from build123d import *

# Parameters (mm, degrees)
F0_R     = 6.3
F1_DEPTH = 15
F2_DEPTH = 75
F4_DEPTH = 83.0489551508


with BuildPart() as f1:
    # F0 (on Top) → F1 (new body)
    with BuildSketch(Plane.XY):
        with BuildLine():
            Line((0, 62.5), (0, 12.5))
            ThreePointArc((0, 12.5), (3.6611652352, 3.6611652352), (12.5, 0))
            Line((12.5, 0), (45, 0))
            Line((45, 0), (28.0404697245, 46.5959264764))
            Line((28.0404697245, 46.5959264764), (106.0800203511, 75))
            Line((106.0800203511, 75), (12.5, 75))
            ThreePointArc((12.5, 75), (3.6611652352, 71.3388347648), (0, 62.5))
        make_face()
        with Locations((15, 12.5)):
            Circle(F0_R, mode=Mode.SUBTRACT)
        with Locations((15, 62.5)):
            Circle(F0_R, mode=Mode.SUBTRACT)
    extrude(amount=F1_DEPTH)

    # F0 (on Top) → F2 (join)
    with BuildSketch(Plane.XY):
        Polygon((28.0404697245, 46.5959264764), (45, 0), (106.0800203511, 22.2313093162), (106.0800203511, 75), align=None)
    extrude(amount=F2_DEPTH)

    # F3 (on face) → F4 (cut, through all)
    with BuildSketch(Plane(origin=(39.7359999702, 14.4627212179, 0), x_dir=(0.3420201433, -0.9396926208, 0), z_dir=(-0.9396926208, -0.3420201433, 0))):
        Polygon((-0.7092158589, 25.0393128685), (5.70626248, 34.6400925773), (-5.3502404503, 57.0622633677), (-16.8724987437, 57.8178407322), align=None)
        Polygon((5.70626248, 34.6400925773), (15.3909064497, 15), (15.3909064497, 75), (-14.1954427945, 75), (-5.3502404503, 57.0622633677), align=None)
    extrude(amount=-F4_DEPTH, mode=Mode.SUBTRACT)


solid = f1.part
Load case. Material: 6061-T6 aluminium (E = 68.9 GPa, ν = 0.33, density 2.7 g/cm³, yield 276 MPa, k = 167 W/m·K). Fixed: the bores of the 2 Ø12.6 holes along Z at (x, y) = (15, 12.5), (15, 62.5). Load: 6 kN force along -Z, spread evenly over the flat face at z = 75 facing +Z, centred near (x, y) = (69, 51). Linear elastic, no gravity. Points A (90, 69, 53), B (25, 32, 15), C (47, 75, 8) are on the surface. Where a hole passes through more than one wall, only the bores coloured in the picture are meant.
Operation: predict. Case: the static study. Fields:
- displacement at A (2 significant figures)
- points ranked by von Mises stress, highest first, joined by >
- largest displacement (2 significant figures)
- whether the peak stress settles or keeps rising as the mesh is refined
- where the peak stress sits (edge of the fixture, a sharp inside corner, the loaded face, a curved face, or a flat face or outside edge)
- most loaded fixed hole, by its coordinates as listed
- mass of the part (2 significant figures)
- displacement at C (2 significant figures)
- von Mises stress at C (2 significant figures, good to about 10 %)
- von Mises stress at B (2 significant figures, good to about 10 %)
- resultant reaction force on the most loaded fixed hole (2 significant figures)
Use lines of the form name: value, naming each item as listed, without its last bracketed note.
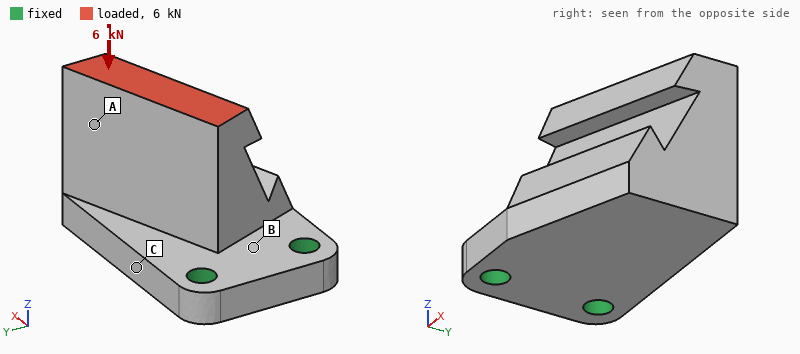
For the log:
displacement at A: 0.35 mm
points ranked by von Mises stress, highest first, joined by >: B > C > A
largest displacement: 0.47 mm
whether the peak stress settles or keeps rising as the mesh is refined: keeps rising
where the peak stress sits: edge of the fixture
most loaded fixed hole, by its coordinates as listed: (15, 62.5)
mass of the part: 650 g
displacement at C: 0.087 mm
von Mises stress at C: 33 MPa
von Mises stress at B: 59 MPa
resultant reaction force on the most loaded fixed hole: 4.5 kN
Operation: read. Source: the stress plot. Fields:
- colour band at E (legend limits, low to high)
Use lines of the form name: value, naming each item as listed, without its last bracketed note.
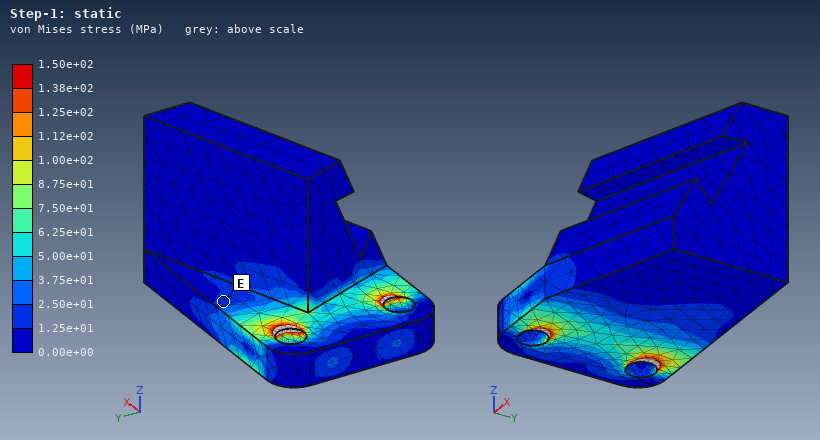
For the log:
colour band at E: 1.25e+01 to 2.50e+01 MPa
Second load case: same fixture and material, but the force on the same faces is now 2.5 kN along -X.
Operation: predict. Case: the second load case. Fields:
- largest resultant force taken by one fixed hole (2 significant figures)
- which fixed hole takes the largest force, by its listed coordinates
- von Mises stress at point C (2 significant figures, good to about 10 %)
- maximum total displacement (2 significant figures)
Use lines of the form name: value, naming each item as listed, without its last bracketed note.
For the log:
largest resultant force taken by one fixed hole: 2.0 kN
which fixed hole takes the largest force, by its listed coordinates: (15, 62.5)
von Mises stress at point C: 13 MPa
maximum total displacement: 0.32 mm
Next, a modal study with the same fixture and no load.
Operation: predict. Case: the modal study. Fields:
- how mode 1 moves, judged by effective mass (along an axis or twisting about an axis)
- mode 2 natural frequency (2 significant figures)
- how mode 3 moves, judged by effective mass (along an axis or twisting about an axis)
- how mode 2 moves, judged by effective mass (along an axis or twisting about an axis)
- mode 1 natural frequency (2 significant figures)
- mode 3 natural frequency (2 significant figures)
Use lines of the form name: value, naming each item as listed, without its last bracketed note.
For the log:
how mode 1 moves, judged by effective mass: along Z
mode 2 natural frequency: 2300 Hz
how mode 3 moves, judged by effective mass: along Y
how mode 2 moves, judged by effective mass: along Y
mode 1 natural frequency: 910 Hz
mode 3 natural frequency: 4600 Hz
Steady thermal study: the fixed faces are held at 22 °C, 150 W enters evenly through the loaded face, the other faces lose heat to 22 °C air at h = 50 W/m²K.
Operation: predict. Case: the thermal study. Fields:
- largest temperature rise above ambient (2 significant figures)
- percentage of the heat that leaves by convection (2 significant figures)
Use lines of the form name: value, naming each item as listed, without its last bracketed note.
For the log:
largest temperature rise above ambient: 51 K
percentage of the heat that leaves by convection: 25 %
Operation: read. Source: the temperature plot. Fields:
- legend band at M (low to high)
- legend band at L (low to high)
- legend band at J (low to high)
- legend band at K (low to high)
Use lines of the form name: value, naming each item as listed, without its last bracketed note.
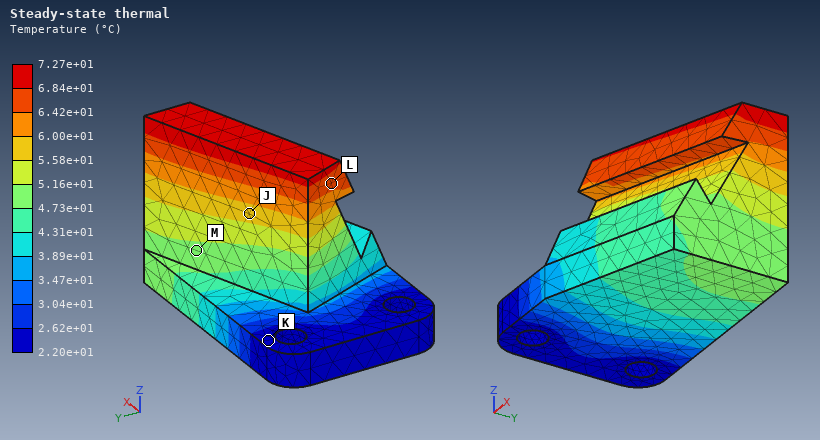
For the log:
legend band at M: 4.73e+01 to 5.16e+01 °C
legend band at L: 6.42e+01 to 6.84e+01 °C
legend band at J: 5.58e+01 to 6.00e+01 °C
legend band at K: 2.20e+01 to 2.62e+01 °C
